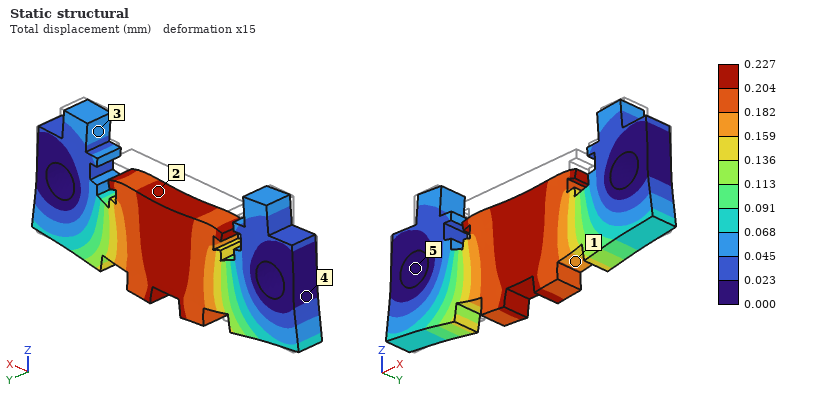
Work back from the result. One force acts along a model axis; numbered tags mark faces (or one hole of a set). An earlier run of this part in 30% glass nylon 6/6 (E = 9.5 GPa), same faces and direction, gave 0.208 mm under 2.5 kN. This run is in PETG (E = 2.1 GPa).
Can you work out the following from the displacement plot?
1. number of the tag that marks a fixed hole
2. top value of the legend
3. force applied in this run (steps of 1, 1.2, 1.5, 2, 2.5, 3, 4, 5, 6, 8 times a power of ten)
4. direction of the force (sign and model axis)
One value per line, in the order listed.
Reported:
5
0.227 mm
600 N
-Z
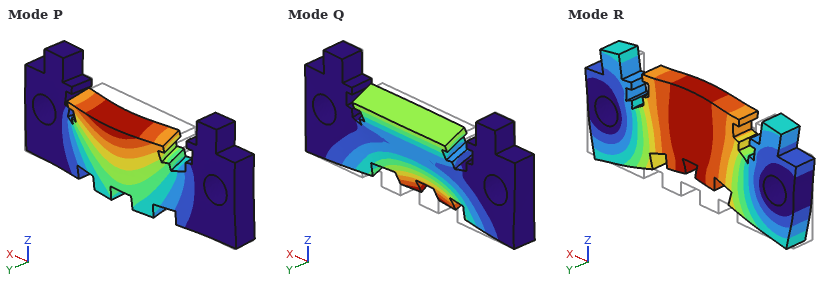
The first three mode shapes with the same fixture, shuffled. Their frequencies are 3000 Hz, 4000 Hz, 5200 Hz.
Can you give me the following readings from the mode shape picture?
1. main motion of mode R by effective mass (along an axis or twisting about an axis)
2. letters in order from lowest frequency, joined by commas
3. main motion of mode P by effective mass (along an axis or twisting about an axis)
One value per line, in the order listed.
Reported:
along Z
P, Q, R
along Y
